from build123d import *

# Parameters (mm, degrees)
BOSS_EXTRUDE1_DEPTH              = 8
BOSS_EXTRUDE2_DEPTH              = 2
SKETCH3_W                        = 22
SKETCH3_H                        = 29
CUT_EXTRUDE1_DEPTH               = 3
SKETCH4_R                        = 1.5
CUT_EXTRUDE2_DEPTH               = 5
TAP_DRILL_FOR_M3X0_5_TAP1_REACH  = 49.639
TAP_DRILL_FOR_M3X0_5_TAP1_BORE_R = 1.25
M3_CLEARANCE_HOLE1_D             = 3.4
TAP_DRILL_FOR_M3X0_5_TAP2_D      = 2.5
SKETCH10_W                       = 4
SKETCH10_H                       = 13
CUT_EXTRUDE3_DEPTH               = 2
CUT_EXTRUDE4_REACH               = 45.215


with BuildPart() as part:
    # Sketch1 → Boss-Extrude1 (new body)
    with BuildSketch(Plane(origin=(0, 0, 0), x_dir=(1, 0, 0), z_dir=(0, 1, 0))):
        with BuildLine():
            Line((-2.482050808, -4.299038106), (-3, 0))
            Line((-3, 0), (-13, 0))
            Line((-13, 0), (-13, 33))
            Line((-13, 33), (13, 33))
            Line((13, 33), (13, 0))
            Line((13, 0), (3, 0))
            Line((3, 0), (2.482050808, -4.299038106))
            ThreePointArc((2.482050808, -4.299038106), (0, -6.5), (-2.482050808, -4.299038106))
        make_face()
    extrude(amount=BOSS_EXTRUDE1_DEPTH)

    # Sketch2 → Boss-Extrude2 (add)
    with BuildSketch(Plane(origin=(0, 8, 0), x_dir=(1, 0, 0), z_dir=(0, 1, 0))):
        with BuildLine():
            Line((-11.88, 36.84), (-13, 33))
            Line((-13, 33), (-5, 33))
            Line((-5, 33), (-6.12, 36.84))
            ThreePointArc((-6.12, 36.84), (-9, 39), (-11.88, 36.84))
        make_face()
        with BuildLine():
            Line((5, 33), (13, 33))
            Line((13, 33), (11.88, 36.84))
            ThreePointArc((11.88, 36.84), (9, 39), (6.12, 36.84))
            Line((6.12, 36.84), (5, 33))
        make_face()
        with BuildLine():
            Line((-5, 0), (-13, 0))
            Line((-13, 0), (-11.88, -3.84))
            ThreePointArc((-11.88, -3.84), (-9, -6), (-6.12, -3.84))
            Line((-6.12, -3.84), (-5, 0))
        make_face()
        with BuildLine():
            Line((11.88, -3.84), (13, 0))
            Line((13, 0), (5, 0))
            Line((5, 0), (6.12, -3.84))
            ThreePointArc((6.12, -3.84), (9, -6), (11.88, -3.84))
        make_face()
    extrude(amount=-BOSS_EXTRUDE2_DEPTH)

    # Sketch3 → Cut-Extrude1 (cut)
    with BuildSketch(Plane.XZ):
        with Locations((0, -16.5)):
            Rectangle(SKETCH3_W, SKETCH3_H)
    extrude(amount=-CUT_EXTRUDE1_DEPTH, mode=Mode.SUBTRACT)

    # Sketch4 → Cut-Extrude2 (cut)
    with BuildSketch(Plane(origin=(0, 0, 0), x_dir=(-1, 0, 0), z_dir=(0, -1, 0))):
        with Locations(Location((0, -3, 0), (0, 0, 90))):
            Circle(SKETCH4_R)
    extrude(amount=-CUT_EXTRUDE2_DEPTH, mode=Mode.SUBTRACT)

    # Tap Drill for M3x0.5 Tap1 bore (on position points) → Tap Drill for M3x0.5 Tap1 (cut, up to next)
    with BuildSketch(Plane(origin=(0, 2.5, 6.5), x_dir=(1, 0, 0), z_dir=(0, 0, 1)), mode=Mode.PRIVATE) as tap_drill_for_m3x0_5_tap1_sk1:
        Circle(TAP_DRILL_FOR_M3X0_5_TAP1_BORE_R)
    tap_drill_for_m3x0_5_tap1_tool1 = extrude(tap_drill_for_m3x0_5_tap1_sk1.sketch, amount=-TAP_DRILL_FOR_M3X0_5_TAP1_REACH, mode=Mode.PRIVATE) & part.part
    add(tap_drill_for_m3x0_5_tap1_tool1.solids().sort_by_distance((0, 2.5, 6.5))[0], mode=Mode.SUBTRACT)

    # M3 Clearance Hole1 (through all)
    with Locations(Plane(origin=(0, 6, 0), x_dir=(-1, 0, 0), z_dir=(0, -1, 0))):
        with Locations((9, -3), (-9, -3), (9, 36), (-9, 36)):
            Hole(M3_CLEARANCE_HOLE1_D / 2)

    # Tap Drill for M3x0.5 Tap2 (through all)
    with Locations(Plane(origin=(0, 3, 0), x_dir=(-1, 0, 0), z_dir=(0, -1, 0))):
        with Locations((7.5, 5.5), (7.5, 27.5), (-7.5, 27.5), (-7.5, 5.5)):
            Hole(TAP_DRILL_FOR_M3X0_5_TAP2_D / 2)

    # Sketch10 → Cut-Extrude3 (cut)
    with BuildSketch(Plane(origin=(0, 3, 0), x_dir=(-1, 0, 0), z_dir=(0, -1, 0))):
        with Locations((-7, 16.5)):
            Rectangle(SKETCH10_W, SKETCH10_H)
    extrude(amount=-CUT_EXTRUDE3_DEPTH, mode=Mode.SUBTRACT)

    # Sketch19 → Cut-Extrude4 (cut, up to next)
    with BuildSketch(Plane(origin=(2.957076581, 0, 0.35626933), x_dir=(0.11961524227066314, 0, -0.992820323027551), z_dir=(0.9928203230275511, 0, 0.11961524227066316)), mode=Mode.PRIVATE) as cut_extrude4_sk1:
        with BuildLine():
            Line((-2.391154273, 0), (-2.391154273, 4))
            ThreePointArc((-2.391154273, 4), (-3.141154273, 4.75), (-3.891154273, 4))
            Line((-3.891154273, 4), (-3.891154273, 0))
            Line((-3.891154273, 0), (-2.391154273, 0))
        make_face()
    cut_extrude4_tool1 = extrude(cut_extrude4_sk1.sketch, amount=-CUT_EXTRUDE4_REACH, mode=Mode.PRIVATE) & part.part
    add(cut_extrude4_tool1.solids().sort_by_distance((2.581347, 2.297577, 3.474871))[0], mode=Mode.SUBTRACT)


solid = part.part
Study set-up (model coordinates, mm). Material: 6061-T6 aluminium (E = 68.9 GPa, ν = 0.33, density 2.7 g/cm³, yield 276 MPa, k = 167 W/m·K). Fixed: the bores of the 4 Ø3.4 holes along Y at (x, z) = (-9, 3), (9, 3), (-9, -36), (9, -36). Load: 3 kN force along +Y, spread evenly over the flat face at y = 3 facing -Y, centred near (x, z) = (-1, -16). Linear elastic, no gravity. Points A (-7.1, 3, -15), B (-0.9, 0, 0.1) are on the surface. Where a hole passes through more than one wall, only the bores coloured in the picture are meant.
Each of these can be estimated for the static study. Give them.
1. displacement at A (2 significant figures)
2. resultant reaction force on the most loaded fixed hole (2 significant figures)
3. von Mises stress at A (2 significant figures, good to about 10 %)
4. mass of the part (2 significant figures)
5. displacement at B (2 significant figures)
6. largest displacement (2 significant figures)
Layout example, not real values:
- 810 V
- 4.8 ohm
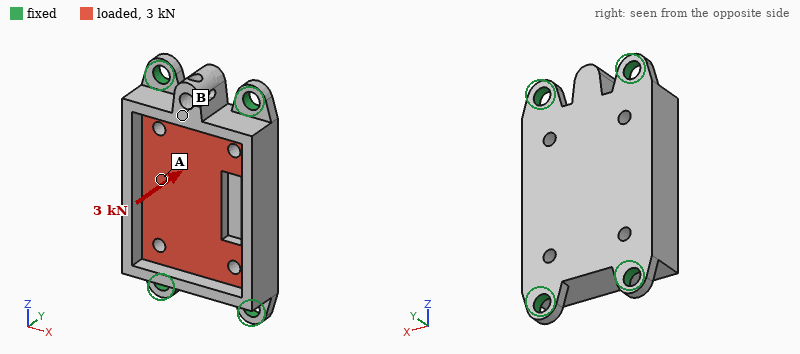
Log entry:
- 54 µm
- 1.2 kN
- 65 MPa
- 14 g
- 25 µm
- 55 µm
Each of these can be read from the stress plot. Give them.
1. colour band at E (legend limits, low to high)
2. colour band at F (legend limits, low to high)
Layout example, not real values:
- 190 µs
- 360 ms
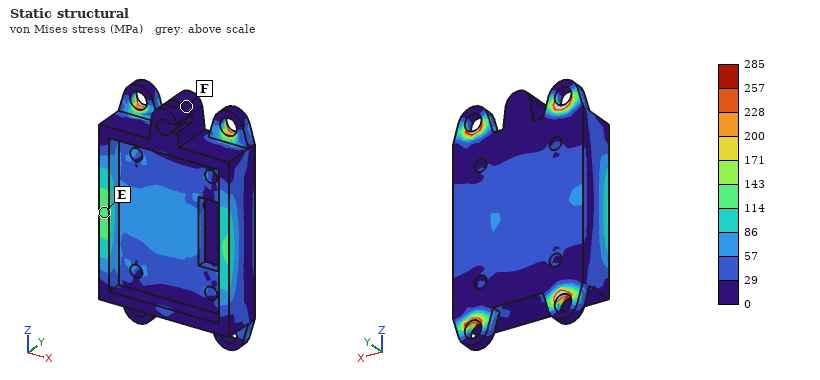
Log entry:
- 114 to 143 MPa
- 0 to 29 MPa
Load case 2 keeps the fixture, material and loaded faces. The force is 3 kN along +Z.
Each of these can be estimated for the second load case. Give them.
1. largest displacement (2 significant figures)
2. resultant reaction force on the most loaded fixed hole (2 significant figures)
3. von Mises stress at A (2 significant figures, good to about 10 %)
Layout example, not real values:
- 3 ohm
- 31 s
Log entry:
- 9.1 µm
- 820 N
- 11 MPa
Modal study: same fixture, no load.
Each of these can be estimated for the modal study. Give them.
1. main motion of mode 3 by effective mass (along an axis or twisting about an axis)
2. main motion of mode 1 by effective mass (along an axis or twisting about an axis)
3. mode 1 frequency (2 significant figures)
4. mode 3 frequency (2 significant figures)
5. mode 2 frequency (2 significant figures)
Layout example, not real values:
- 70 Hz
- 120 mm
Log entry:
- along X
- along Y
- 12 kHz
- 22 kHz
- 16 kHz
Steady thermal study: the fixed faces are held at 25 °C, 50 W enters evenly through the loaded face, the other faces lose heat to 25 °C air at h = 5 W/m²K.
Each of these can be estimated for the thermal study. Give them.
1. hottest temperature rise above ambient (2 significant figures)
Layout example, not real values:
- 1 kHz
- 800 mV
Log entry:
- 29 K
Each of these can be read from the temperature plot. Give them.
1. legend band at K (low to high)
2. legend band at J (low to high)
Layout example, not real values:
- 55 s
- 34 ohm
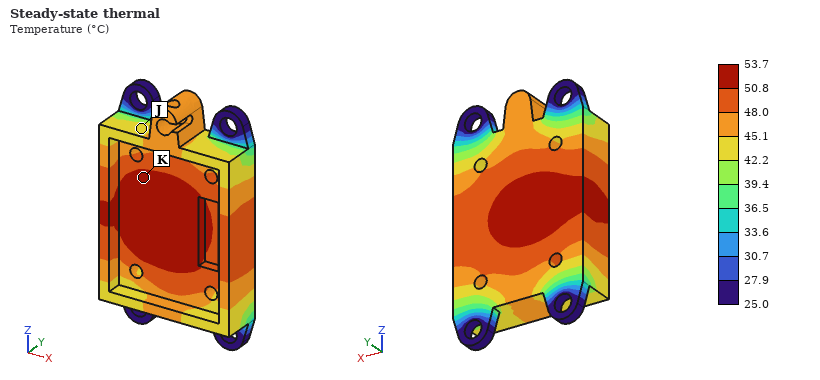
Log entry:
- 50.8 to 53.7 °C
- 42.2 to 45.1 °C
